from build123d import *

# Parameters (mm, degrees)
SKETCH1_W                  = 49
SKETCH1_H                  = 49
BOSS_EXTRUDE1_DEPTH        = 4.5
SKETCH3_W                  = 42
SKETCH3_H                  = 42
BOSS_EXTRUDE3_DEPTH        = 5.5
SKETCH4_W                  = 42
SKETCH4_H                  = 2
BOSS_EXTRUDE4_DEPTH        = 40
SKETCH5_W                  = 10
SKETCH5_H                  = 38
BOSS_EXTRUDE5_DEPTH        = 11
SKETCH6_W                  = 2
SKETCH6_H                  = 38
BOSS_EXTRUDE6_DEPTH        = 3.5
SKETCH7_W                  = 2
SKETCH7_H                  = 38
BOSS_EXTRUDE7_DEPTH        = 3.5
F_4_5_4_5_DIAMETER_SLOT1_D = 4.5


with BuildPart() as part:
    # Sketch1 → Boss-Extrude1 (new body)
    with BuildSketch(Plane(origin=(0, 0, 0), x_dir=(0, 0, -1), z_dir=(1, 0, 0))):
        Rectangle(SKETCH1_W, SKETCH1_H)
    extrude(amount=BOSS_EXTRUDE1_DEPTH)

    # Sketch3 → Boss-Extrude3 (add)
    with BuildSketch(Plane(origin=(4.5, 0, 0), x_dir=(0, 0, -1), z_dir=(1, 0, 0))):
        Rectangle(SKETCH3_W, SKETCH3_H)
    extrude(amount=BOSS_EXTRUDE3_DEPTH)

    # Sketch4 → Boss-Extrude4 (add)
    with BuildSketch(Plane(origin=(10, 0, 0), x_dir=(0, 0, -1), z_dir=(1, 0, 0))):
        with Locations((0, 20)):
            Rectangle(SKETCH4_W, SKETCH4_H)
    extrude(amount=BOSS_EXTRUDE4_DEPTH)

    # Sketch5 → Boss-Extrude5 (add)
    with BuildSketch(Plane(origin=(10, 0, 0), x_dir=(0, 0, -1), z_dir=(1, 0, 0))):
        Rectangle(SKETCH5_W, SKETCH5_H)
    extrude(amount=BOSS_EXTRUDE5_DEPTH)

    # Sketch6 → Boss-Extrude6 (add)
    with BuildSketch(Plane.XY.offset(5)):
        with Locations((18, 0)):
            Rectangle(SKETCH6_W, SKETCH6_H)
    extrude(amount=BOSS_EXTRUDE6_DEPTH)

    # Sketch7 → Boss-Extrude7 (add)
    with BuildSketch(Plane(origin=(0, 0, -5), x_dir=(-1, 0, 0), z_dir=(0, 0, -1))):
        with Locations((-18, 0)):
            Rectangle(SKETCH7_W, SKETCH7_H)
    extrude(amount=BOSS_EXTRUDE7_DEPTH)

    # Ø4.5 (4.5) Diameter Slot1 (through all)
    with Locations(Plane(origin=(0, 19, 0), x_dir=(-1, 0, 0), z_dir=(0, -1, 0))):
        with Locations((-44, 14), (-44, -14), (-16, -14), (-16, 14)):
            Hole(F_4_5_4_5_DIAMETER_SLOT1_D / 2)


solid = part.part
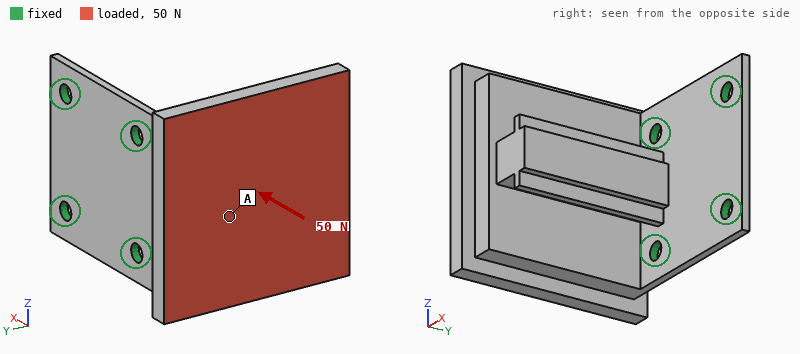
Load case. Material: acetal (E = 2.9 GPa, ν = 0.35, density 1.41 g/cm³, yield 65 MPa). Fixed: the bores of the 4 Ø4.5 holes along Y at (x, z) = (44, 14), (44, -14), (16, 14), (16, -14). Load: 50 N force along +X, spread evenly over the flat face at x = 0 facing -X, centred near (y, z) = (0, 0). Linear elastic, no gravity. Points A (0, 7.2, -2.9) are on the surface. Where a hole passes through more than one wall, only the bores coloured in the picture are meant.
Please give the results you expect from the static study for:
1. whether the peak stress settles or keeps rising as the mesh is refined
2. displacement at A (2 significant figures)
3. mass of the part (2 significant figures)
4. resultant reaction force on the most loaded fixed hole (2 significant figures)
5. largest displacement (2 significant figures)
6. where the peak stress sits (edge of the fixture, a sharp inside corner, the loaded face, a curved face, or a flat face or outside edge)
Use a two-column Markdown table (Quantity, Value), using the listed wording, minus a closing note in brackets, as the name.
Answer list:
| Quantity | Value |
|---|---|
| whether the peak stress settles or keeps rising as the mesh is refined | keeps rising |
| displacement at A | 0.35 mm |
| mass of the part | 40 g |
| resultant reaction force on the most loaded fixed hole | 19 N |
| largest displacement | 0.86 mm |
| where the peak stress sits | edge of the fixture |
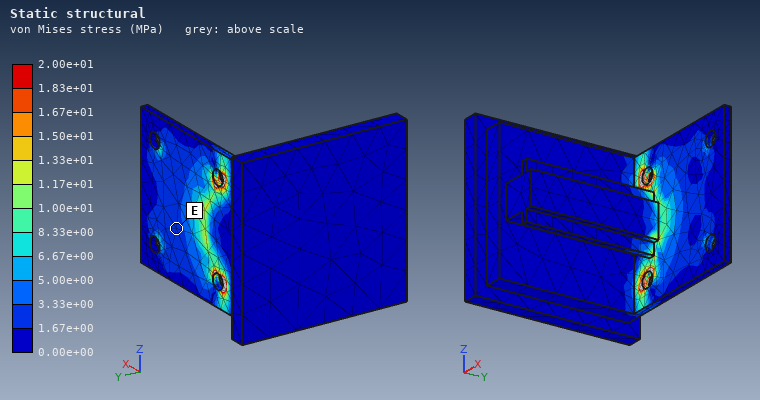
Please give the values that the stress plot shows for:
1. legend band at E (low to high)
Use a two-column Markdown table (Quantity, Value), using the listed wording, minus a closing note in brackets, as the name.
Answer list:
| Quantity | Value |
|---|---|
| legend band at E | 1.67e+00 to 3.33e+00 MPa |
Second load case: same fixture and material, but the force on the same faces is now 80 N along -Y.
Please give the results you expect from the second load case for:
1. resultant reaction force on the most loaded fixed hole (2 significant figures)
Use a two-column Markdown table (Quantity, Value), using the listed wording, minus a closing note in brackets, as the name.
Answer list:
| Quantity | Value |
|---|---|
| resultant reaction force on the most loaded fixed hole | 47 N |
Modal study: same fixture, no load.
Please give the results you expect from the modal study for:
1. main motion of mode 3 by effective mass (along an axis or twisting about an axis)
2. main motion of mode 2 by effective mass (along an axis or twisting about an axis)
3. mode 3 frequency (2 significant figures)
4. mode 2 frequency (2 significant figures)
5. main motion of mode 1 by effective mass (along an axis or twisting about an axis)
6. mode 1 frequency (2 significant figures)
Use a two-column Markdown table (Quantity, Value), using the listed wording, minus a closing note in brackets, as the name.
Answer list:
| Quantity | Value |
|---|---|
| main motion of mode 3 by effective mass | along Y |
| main motion of mode 2 by effective mass | along Z |
| mode 3 frequency | 1600 Hz |
| mode 2 frequency | 750 Hz |
| main motion of mode 1 by effective mass | along X |
| mode 1 frequency | 240 Hz |
